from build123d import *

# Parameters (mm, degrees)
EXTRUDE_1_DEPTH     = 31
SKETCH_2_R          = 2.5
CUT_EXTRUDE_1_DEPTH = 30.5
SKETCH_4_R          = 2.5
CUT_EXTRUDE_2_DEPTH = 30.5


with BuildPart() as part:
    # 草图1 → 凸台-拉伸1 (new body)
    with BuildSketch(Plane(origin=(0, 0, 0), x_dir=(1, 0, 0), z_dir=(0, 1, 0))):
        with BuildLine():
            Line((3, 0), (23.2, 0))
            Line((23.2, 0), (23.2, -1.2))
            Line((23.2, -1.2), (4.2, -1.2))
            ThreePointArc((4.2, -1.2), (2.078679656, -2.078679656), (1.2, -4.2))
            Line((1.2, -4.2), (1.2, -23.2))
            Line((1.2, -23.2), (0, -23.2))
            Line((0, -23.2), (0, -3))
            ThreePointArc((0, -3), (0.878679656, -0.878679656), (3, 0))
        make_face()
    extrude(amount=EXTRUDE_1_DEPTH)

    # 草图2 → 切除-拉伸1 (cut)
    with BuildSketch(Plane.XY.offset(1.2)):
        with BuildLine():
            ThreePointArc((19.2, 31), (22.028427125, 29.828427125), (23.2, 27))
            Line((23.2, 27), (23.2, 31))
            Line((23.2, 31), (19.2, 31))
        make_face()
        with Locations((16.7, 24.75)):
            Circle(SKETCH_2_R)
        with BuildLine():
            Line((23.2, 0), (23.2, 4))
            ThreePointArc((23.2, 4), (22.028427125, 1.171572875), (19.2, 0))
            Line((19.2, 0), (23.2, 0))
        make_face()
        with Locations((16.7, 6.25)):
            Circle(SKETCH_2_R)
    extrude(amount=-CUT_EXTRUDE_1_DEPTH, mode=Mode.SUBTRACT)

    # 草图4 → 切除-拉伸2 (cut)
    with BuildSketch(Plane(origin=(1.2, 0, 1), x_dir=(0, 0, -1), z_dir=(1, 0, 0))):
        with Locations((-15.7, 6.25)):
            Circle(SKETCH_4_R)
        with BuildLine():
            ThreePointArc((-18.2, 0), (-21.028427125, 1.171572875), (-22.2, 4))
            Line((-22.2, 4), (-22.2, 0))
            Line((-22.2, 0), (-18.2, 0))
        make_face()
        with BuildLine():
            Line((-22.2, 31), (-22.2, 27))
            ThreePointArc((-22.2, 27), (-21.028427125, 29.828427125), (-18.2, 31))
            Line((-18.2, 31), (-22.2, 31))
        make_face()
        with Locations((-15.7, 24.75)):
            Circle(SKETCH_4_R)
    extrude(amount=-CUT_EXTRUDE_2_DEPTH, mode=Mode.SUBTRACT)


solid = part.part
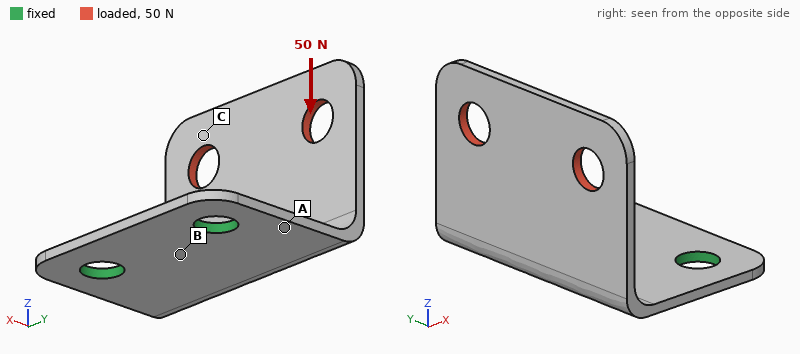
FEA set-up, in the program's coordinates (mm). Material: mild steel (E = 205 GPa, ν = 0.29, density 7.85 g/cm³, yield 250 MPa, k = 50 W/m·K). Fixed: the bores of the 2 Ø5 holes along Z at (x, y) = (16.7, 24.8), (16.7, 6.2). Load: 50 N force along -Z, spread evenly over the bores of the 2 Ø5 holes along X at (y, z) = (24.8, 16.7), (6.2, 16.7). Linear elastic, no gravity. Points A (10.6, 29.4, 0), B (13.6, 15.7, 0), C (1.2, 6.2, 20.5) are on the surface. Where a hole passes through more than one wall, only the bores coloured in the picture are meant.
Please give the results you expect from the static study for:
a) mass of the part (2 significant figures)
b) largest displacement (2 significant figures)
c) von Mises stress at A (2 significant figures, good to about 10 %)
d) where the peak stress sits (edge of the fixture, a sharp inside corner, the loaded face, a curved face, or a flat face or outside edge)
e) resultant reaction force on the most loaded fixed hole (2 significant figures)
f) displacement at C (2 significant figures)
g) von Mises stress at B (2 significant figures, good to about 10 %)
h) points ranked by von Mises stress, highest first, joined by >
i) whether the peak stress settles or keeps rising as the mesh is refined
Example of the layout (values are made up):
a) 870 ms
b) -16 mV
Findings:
a) 12 g
b) 0.14 mm
c) 69 MPa
d) edge of the fixture
e) 25 N
f) 0.12 mm
g) 48 MPa
h) A > B > C
i) keeps rising
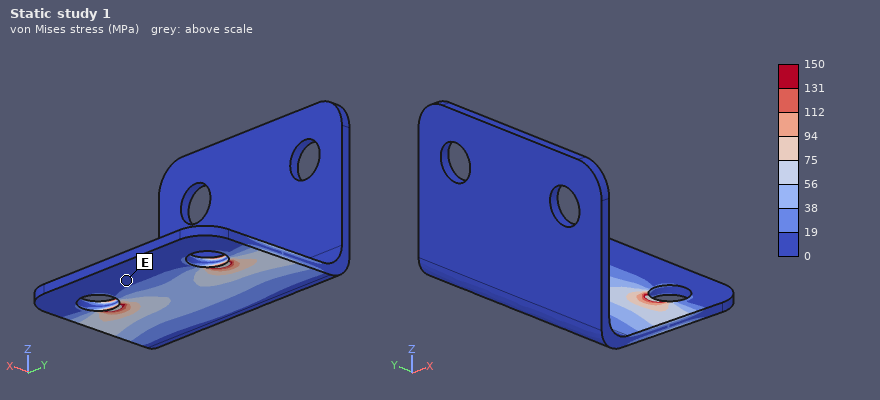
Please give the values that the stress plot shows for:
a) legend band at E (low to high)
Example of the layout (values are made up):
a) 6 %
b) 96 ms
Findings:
a) 0 to 19 MPa
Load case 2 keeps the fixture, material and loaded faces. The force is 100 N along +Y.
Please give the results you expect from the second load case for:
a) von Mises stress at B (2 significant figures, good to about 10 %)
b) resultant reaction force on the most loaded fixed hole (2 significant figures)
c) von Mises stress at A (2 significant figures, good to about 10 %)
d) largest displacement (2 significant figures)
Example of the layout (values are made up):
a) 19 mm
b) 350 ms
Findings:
a) 23 MPa
b) 110 N
c) 92 MPa
d) 0.15 mm
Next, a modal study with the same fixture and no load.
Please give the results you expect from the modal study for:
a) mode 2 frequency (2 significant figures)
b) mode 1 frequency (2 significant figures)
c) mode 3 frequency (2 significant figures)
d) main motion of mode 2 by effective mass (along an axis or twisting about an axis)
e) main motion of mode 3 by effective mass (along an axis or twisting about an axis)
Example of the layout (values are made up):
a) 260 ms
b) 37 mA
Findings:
a) 2100 Hz
b) 1100 Hz
c) 3300 Hz
d) along Y
e) along Z
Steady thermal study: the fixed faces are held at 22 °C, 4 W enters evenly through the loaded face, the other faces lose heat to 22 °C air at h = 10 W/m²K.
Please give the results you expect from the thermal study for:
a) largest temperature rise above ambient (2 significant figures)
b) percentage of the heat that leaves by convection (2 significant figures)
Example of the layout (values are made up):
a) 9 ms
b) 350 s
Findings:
a) 61 K
b) 18 %
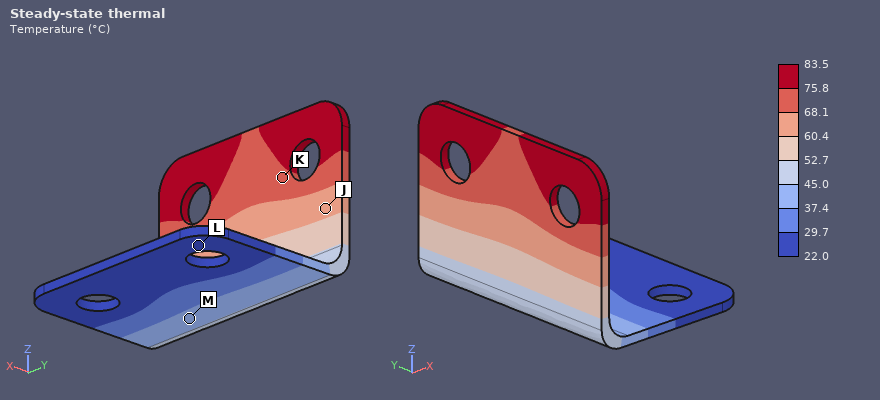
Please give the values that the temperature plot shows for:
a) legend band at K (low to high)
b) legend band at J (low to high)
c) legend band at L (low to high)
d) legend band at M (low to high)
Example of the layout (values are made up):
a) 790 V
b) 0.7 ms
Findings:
a) 68.1 to 75.8 °C
b) 60.4 to 68.1 °C
c) 22.0 to 29.7 °C
d) 37.4 to 45.0 °C
